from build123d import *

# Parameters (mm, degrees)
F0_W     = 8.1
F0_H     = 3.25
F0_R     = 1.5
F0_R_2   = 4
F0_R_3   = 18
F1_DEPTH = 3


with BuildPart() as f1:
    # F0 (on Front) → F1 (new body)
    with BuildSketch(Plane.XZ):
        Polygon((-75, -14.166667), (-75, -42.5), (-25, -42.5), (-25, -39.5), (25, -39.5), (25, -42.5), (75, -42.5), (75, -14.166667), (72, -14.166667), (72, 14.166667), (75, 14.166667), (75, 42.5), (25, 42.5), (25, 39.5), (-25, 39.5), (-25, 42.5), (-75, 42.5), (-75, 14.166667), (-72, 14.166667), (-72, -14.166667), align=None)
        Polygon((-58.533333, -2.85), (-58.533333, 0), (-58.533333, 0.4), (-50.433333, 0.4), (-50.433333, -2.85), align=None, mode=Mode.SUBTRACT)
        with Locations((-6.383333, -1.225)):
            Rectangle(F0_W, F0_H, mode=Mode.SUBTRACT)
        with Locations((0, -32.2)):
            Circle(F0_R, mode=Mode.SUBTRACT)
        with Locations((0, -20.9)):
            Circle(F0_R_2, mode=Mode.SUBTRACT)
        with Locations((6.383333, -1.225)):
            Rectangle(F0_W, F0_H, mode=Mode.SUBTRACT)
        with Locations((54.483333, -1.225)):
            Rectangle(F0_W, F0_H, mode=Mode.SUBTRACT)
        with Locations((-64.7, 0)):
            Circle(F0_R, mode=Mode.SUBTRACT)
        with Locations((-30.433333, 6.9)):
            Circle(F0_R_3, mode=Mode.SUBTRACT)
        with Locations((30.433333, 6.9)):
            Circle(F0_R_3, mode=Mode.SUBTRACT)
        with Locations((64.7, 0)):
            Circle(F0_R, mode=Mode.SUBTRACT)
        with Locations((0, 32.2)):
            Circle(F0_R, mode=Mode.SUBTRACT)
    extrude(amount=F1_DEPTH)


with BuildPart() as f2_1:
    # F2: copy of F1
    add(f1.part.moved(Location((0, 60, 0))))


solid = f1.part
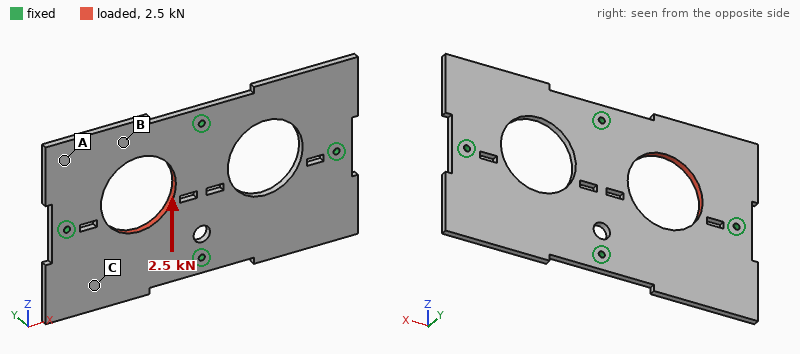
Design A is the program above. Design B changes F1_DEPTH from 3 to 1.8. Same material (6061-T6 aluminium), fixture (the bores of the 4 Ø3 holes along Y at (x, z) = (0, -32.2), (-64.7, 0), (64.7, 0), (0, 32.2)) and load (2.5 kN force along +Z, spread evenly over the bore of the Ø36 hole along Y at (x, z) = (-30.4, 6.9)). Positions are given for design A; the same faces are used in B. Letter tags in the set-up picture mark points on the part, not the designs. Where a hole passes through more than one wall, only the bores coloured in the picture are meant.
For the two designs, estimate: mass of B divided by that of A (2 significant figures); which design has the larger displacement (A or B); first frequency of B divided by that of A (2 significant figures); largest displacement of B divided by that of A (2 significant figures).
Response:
0.60
B
0.63
1.7
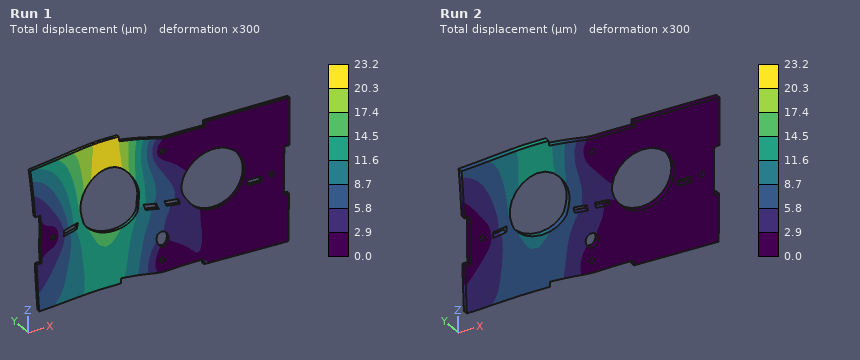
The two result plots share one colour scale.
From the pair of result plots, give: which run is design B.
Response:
Run 1
